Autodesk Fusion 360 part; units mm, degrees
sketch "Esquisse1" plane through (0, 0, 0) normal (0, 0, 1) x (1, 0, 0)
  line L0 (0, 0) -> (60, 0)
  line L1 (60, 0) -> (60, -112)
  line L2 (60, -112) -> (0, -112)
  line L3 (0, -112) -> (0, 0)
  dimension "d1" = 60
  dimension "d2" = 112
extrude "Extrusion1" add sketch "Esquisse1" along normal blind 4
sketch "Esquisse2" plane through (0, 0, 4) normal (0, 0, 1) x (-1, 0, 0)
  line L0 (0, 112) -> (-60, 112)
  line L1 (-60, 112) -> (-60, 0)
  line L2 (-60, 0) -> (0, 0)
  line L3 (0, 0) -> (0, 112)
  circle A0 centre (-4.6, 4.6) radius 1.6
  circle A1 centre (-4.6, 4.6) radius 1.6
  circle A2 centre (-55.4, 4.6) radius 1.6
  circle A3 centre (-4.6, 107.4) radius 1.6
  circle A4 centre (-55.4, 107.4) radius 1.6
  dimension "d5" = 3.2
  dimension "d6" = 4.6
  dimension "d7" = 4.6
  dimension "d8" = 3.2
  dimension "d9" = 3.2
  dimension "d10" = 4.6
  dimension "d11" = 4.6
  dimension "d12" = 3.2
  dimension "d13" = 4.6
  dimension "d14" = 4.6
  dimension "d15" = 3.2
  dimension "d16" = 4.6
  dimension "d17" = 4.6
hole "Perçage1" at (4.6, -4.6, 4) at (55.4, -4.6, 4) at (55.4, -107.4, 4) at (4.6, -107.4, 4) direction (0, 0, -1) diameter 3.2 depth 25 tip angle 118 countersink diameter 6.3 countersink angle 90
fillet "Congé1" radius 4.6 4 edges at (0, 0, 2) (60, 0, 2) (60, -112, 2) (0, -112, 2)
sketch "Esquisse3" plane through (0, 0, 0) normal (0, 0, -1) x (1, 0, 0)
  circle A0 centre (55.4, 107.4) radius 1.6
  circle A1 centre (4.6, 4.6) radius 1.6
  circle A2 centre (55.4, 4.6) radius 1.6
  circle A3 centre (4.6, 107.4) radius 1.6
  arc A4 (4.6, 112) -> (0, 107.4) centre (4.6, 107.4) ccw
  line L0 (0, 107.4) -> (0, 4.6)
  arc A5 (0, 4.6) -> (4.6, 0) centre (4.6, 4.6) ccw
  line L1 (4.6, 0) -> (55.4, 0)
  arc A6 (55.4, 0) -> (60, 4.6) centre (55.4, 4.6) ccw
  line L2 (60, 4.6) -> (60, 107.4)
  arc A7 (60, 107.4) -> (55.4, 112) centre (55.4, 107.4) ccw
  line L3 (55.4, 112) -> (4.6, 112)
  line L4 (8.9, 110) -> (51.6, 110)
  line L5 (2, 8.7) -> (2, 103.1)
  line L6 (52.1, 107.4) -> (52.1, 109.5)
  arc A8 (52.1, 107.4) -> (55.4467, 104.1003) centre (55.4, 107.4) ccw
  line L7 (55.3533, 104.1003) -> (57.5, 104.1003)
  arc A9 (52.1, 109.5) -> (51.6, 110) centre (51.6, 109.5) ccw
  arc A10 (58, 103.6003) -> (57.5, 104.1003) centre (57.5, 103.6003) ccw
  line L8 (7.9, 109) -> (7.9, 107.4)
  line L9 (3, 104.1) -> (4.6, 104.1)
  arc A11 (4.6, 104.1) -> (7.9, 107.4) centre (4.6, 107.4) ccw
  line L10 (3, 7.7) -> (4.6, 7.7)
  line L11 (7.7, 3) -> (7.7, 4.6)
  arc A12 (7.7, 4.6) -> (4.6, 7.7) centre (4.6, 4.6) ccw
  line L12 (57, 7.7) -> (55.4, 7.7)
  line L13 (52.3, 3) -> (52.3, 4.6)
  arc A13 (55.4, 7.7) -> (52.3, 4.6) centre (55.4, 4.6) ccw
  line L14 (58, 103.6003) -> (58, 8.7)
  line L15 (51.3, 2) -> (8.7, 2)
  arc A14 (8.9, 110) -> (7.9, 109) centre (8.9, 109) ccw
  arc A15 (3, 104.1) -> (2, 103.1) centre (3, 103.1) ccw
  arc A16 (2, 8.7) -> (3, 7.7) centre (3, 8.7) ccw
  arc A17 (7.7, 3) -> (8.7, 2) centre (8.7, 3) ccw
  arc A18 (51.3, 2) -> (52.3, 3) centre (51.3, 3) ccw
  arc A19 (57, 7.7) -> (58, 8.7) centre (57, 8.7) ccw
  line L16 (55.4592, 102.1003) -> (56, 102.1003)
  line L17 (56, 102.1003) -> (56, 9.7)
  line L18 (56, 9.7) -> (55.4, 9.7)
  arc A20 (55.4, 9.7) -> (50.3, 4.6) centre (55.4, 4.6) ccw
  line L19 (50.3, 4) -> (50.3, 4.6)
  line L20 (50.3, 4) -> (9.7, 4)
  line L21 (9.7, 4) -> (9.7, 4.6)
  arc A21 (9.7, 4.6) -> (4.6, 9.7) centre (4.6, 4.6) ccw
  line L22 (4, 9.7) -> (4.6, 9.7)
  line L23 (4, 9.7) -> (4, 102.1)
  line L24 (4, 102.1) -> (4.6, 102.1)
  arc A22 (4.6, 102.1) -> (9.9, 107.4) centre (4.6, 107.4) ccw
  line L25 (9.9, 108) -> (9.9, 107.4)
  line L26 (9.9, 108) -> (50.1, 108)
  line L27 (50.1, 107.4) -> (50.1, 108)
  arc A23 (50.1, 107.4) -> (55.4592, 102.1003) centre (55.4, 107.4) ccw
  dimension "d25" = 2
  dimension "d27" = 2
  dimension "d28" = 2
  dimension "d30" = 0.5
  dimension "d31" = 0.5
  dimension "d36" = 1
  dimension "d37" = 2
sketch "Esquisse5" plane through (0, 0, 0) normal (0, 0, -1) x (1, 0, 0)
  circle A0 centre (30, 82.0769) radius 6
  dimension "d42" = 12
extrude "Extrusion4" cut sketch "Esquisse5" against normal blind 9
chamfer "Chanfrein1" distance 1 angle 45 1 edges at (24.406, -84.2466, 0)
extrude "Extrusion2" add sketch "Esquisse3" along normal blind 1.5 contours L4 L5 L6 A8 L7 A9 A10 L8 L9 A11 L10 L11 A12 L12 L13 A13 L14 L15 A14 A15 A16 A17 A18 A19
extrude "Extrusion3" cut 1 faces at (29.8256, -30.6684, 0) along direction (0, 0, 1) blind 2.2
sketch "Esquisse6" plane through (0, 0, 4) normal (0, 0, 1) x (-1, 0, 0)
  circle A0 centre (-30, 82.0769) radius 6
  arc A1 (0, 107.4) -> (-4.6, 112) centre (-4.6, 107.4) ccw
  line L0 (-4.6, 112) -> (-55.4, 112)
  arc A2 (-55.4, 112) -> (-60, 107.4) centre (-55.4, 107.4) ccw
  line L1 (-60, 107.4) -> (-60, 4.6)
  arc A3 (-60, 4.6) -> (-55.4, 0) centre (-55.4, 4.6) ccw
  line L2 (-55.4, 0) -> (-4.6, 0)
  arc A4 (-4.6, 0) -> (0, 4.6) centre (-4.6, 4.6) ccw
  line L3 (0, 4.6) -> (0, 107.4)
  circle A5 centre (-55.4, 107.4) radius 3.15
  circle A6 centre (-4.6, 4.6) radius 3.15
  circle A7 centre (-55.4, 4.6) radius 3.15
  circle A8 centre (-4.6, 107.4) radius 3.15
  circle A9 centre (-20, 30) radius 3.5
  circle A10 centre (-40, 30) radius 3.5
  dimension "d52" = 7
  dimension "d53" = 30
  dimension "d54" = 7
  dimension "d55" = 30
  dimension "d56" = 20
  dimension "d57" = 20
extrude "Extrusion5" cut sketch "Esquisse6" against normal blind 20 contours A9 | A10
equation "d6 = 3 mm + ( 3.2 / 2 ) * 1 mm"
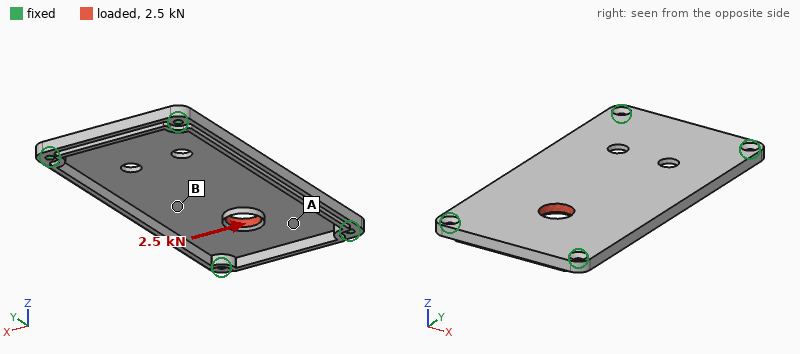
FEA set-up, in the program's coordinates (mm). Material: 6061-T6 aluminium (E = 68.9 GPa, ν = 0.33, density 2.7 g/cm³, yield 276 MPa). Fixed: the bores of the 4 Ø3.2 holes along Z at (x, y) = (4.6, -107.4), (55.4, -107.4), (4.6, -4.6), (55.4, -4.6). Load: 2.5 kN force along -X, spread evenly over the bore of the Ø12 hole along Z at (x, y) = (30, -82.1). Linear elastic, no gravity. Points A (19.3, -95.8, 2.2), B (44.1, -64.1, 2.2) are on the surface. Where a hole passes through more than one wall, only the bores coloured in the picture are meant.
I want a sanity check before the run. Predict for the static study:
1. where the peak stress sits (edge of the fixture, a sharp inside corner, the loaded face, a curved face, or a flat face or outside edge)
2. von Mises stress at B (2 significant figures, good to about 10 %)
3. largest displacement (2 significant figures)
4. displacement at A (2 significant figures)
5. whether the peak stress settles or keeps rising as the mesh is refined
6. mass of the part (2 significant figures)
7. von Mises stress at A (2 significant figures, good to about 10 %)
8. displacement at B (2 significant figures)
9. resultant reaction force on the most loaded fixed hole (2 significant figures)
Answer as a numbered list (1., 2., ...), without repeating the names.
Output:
1. edge of the fixture
2. 15 MPa
3. 61 µm
4. 24 µm
5. keeps rising
6. 42 g
7. 44 MPa
8. 47 µm
9. 1.1 kN
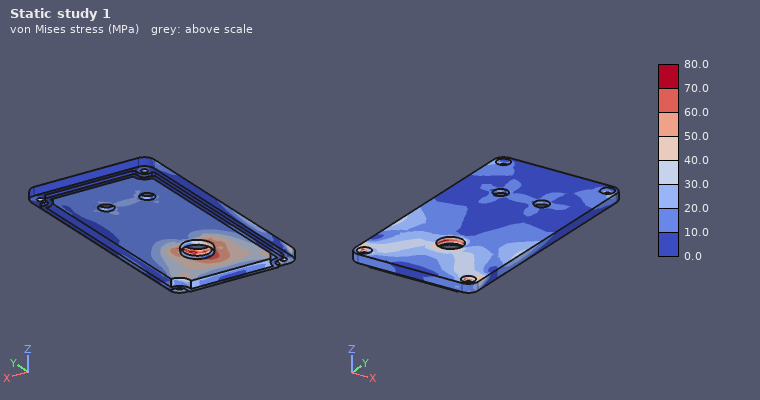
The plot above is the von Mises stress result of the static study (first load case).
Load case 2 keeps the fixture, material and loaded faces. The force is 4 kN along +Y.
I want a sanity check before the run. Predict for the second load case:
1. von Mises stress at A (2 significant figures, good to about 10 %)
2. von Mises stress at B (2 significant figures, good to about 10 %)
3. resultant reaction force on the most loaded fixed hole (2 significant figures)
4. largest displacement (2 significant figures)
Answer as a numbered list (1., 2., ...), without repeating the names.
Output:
1. 47 MPa
2. 28 MPa
3. 1.4 kN
4. 68 µm
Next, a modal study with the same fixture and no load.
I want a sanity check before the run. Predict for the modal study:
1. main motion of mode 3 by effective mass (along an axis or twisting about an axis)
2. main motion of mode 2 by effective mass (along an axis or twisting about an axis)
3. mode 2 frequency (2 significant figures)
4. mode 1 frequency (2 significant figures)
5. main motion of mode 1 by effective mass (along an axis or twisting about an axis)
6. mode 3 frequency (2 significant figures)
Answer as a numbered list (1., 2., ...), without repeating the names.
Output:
1. twisting about X
2. twisting about Y
3. 2200 Hz
4. 1500 Hz
5. along Z
6. 3400 Hz
